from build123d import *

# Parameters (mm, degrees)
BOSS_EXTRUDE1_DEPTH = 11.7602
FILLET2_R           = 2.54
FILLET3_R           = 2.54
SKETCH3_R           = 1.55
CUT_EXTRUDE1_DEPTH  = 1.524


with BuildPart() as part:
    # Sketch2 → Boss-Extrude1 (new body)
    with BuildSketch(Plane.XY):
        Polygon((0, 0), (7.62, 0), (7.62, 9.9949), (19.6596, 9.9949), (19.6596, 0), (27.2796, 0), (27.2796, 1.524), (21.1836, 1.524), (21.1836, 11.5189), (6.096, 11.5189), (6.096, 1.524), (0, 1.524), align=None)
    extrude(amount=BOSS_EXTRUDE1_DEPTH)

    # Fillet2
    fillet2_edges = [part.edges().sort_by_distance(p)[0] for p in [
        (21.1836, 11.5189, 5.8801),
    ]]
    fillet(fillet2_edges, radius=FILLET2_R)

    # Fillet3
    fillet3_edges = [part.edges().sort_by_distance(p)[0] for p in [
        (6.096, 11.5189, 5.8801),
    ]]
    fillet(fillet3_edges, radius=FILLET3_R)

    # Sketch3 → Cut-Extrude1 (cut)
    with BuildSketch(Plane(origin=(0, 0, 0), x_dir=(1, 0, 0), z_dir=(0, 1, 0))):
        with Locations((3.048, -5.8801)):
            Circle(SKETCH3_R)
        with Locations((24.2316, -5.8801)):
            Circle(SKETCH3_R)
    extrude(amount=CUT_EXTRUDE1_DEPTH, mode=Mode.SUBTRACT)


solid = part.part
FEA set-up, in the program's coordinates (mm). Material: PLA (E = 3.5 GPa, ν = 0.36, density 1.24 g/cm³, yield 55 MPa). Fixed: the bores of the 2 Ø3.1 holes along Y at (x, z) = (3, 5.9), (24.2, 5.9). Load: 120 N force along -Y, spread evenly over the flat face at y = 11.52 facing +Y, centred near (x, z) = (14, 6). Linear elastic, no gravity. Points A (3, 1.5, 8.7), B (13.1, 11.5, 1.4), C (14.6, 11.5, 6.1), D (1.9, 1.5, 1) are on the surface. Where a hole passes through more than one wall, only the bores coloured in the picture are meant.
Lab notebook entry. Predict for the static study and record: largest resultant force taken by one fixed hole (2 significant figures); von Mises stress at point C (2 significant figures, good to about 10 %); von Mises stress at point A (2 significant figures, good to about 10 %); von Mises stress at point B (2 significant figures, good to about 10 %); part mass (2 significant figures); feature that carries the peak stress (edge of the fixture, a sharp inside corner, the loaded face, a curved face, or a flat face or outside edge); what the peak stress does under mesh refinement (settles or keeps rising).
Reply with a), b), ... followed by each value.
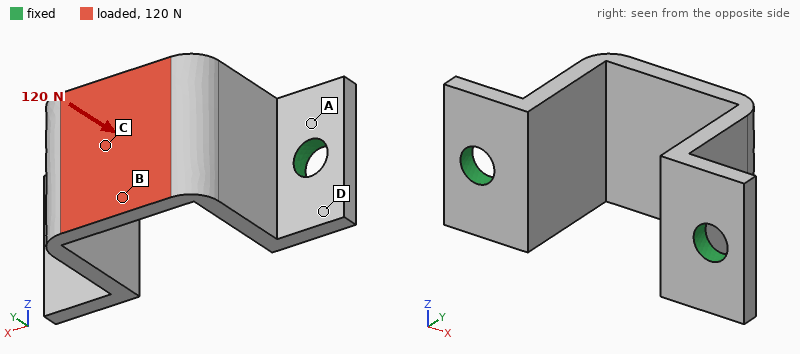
a) 64 N
b) 25 MPa
c) 5.3 MPa
d) 28 MPa
e) 0.98 g
f) edge of the fixture
g) keeps rising
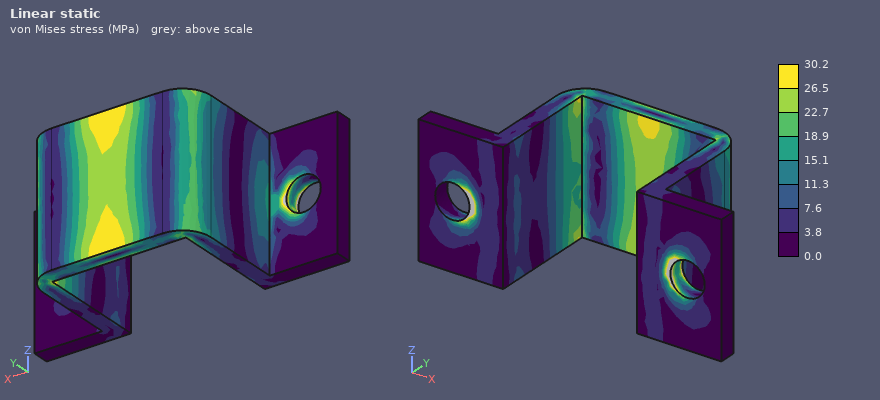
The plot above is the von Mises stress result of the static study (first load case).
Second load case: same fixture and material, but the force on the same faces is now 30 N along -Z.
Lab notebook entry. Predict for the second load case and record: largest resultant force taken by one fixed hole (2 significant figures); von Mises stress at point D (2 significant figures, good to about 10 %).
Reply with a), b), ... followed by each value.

a) 15 N
b) 6.4 MPa
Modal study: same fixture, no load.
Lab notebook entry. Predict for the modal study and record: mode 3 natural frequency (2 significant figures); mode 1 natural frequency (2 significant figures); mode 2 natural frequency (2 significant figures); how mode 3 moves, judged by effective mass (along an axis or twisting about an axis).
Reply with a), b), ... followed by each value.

a) 4400 Hz
b) 2900 Hz
c) 2900 Hz
d) twisting about Y
